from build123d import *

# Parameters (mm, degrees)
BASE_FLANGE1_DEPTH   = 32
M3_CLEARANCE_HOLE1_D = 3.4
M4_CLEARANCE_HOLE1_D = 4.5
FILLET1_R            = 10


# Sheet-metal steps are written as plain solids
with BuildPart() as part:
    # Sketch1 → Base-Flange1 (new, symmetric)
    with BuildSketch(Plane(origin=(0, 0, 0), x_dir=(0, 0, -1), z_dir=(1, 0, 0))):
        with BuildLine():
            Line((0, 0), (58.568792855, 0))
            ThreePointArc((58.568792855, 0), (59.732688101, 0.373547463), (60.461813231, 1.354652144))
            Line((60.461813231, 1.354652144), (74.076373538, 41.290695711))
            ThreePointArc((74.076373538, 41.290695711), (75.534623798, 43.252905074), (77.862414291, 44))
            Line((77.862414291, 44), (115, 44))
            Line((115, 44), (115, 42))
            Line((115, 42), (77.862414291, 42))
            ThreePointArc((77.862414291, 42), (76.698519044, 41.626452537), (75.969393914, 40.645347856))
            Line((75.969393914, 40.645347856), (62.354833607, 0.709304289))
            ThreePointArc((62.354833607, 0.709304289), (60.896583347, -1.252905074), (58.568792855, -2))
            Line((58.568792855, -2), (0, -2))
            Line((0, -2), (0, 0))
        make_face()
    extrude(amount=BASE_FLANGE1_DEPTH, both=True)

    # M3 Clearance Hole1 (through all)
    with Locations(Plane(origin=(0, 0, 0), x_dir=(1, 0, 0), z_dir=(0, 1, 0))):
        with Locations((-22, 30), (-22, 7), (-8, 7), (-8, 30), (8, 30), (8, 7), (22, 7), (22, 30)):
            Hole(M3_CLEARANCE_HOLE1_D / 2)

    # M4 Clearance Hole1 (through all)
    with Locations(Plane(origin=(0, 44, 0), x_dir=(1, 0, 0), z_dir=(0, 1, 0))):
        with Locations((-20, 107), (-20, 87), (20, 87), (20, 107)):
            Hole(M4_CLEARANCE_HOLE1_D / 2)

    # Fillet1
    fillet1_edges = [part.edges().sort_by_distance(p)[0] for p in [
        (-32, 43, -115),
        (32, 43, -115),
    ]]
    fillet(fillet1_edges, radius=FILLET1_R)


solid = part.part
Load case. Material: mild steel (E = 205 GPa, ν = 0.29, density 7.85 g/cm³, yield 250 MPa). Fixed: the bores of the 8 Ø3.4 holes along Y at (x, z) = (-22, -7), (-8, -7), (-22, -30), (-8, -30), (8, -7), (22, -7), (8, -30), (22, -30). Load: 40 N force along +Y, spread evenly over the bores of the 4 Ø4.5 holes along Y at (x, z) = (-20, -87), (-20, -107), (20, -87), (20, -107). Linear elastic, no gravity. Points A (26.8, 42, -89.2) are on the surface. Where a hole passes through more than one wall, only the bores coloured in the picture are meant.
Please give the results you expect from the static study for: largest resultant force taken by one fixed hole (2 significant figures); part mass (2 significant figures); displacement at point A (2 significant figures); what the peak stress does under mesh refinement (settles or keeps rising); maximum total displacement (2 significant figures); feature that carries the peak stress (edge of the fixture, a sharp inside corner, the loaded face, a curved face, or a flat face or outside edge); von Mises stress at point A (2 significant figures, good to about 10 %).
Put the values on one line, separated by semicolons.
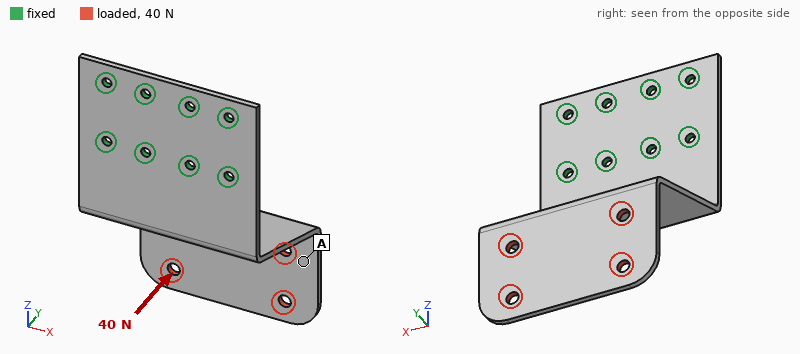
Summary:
16 N; 140 g; 0.60 mm; keeps rising; 0.90 mm; edge of the fixture; 8.4 MPa
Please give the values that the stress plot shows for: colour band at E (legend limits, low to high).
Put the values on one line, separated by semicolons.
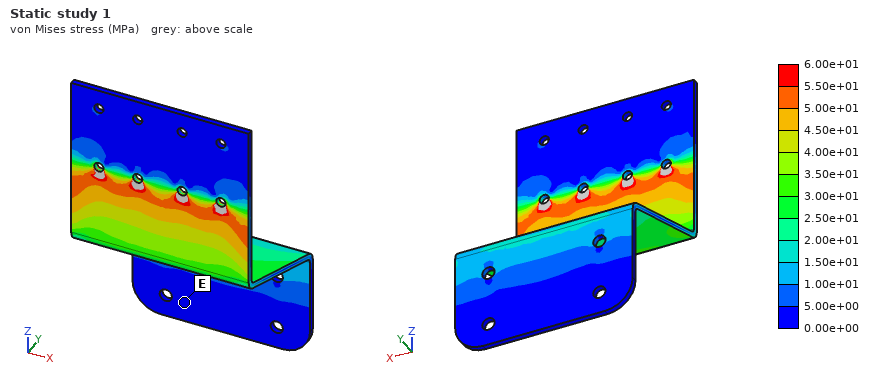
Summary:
0.00e+00 to 5.00e+00 MPa
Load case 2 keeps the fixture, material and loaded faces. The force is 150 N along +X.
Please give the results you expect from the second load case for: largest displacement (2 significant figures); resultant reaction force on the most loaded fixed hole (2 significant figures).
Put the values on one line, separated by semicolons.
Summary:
0.39 mm; 220 N
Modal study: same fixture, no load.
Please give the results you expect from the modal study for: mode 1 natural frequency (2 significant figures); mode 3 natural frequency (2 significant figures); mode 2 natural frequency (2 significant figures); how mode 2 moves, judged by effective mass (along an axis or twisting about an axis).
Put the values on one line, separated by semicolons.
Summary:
160 Hz; 570 Hz; 480 Hz; along X
